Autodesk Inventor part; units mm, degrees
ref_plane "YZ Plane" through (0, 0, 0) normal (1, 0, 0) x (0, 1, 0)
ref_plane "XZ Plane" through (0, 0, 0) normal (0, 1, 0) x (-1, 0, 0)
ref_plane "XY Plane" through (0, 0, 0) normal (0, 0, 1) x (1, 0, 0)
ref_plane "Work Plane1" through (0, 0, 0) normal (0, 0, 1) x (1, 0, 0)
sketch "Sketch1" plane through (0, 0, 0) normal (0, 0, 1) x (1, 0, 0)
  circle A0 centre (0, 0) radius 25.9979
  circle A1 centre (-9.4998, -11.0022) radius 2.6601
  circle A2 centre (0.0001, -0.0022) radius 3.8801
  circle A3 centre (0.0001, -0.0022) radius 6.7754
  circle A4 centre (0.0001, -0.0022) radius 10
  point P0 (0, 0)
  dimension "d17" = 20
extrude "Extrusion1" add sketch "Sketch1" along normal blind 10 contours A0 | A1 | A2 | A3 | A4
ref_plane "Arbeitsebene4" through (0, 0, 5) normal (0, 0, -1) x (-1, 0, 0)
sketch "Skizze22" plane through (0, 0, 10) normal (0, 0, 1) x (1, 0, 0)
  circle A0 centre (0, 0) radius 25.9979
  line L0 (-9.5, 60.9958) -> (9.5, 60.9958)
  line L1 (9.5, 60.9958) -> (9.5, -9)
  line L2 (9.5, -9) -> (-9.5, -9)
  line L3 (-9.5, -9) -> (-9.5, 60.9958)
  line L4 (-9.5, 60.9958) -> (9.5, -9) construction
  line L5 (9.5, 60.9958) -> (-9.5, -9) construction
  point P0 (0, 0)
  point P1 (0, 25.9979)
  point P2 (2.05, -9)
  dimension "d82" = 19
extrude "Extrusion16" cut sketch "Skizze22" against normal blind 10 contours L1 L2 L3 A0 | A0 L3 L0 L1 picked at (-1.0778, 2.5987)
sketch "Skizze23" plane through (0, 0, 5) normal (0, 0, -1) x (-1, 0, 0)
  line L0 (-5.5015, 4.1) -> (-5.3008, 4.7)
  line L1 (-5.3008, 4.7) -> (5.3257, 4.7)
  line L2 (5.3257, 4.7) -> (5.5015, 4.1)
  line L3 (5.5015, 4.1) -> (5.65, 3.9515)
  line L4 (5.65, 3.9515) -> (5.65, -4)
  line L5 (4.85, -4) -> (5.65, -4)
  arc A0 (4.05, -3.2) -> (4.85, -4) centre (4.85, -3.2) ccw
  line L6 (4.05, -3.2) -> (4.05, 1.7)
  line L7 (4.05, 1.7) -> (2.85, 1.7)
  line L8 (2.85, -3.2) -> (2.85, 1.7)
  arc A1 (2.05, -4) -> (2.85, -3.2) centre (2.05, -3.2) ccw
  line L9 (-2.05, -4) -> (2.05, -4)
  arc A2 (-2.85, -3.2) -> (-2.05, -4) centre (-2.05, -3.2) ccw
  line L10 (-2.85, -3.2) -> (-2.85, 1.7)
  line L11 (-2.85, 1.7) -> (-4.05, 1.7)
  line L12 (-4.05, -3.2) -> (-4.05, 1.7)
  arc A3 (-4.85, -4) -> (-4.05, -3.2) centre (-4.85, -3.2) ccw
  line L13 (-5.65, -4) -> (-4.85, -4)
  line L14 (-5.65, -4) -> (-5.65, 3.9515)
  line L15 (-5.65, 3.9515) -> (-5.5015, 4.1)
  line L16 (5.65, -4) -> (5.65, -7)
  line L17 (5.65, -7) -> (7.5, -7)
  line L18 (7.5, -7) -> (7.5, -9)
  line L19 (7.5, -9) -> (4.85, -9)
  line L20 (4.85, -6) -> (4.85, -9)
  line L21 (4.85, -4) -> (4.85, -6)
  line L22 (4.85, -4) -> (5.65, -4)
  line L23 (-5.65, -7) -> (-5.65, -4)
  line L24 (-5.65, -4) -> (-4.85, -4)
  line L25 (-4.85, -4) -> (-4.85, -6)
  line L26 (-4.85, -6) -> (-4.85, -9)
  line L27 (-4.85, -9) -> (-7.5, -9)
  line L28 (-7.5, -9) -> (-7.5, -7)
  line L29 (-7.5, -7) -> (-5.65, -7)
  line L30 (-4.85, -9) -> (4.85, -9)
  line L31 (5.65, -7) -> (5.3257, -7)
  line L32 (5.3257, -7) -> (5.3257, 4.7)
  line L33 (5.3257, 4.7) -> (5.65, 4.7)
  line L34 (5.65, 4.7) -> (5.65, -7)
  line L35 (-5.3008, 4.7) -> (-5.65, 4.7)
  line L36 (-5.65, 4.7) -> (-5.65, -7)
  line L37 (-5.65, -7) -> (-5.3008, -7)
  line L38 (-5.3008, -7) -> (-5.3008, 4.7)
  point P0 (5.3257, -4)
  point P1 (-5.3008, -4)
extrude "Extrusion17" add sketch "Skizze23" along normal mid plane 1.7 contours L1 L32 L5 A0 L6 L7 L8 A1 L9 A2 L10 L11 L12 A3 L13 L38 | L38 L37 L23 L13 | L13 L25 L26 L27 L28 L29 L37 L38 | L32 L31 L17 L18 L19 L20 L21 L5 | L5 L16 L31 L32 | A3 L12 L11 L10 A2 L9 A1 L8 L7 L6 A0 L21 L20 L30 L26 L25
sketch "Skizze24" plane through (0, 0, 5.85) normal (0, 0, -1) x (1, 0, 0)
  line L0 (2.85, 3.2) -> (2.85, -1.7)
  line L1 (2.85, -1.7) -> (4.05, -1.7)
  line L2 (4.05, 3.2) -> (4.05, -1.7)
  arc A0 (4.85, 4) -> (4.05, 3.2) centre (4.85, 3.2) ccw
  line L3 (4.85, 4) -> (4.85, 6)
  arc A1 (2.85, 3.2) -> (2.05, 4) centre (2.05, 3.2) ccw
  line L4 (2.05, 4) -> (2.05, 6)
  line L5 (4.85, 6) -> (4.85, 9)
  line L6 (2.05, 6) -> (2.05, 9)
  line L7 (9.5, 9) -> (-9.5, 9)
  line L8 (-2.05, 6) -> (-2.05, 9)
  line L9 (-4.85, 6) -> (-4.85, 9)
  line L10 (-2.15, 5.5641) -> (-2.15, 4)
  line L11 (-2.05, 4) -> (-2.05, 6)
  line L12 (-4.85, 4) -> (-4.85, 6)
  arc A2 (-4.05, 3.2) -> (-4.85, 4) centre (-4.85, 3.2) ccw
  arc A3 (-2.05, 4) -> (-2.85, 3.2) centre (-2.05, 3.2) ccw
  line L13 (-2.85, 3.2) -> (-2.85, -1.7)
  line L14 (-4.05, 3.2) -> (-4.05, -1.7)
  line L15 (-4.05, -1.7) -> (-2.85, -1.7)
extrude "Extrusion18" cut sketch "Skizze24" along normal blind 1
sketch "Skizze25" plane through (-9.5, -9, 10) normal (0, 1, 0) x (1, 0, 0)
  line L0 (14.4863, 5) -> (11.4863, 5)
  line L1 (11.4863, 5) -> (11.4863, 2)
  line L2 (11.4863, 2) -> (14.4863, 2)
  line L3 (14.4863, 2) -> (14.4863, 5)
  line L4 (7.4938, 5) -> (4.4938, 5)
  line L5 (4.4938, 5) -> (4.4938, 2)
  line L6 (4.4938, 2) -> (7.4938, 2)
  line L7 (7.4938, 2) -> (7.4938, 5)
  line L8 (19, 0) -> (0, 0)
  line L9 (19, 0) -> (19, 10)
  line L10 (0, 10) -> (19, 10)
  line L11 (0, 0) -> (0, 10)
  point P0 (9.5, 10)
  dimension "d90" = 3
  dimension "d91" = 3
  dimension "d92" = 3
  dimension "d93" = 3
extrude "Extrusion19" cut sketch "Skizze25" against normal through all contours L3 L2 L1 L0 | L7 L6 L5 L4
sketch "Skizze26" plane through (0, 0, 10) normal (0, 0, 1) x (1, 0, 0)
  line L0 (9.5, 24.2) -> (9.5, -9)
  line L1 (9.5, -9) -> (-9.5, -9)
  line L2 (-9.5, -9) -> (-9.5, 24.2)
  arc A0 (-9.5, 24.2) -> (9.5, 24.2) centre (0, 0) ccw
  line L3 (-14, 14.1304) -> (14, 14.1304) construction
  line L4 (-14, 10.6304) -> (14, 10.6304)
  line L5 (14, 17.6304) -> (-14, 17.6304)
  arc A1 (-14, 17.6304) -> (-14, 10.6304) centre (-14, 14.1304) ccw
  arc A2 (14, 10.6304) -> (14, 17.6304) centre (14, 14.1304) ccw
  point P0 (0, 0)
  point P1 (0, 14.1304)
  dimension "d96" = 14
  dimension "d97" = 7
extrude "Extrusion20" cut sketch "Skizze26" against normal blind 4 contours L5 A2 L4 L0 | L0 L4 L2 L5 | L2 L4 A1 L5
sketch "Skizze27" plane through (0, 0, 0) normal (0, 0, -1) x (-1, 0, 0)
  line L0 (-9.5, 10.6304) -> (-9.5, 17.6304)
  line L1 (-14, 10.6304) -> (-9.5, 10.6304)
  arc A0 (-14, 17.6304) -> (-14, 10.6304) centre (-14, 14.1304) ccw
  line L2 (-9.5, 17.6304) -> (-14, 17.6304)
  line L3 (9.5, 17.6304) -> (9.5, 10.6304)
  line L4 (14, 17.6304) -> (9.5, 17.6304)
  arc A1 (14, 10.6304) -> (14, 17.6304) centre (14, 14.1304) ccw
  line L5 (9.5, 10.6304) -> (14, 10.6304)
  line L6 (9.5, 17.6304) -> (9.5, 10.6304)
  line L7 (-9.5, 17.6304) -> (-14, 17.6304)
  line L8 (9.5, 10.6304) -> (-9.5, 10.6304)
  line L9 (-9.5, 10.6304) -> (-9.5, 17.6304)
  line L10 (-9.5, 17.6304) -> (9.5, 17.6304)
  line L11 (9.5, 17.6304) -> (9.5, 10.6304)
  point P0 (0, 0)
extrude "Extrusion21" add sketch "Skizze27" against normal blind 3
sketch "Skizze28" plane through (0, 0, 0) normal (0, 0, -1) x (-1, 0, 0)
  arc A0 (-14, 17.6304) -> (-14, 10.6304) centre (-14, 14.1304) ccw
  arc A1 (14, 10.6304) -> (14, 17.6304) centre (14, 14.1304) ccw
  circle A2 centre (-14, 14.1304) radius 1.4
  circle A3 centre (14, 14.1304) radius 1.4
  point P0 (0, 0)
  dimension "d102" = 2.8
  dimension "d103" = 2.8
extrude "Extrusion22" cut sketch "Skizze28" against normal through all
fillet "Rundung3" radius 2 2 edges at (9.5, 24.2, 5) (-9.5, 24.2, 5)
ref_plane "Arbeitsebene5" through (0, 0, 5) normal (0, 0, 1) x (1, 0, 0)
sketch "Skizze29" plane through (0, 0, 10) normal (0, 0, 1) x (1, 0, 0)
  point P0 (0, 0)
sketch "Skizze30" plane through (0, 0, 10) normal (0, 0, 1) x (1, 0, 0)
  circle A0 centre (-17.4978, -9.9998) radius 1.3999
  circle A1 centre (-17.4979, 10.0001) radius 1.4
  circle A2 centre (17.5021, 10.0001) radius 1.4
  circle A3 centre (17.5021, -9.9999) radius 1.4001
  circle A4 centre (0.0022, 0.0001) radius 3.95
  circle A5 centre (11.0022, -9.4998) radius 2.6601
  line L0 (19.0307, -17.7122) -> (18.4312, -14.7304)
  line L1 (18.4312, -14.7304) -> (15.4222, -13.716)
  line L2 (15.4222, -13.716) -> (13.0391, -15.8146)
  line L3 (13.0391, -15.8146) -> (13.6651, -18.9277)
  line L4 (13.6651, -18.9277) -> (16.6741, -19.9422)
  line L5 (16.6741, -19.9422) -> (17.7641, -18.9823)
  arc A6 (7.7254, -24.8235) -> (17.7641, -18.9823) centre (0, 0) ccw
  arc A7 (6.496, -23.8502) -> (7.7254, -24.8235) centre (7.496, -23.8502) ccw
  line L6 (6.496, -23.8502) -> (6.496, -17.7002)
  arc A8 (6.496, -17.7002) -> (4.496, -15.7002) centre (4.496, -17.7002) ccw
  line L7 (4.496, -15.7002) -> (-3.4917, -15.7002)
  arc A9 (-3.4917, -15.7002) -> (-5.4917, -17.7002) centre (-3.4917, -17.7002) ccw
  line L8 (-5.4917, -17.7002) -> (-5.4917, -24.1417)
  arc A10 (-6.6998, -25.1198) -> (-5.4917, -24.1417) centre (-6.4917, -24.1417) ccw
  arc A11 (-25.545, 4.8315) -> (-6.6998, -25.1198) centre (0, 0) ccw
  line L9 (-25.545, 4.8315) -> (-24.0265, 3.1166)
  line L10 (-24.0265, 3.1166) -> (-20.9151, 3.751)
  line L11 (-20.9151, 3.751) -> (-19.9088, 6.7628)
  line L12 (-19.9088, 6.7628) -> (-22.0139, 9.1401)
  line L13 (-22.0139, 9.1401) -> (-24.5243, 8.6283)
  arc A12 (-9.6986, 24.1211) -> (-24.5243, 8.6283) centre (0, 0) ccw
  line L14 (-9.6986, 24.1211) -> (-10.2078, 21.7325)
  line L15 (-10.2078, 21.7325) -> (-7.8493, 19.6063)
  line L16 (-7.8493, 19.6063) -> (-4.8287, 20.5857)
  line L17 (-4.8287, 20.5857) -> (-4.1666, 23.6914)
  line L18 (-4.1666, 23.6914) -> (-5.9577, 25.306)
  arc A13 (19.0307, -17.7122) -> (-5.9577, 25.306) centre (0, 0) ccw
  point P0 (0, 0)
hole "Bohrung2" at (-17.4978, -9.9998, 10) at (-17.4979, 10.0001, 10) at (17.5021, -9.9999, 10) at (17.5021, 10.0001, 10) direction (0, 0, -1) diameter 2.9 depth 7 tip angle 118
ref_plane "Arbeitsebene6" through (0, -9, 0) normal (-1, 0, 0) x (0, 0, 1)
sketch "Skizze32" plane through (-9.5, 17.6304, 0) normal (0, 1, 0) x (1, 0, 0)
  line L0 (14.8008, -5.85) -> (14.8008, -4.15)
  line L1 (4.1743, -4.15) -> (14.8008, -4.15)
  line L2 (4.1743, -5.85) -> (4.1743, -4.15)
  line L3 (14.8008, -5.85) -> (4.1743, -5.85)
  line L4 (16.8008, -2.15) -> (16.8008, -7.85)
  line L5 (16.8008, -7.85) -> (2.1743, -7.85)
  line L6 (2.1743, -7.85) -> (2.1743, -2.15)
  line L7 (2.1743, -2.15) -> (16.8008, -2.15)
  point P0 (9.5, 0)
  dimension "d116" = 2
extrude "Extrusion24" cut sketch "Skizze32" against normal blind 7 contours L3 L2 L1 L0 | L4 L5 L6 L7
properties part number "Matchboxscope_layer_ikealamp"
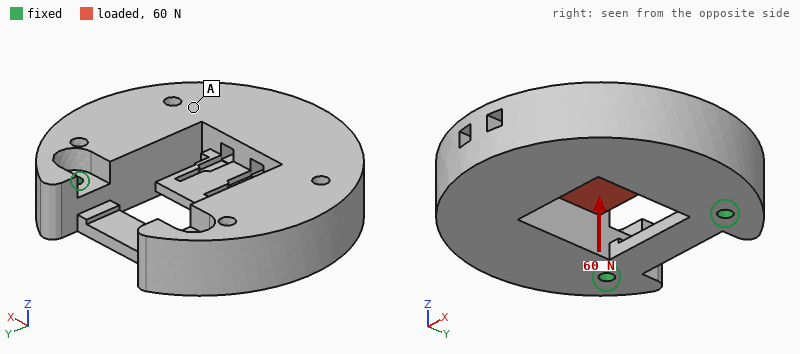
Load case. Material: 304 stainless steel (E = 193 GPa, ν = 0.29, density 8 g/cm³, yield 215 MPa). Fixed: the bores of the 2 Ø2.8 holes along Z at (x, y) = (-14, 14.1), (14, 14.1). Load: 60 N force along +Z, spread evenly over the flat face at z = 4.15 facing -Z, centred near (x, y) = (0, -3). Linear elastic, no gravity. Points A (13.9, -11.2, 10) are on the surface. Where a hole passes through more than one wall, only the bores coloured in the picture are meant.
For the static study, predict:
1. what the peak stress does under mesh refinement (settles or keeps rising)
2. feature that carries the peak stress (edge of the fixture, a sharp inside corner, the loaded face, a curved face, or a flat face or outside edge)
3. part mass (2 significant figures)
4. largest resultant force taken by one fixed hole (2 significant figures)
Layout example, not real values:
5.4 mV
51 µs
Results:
keeps rising
a sharp inside corner
110 g
30 N
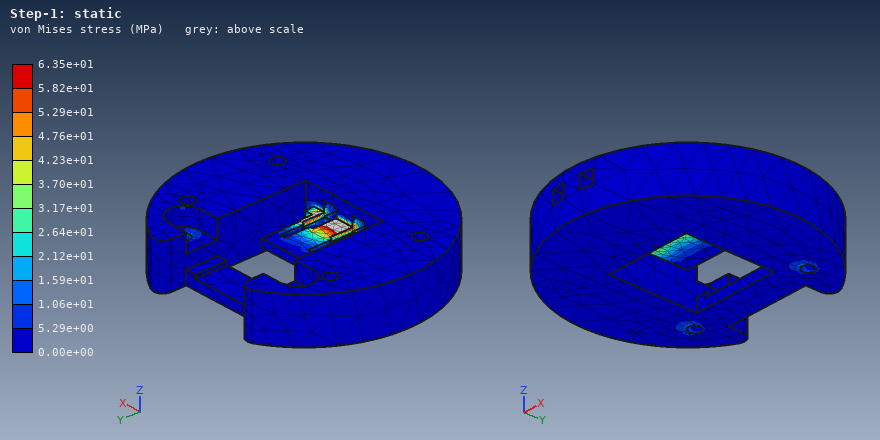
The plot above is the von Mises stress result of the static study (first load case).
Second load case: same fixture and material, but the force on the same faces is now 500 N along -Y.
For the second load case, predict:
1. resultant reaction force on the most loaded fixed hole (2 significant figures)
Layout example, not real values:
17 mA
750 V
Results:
250 N
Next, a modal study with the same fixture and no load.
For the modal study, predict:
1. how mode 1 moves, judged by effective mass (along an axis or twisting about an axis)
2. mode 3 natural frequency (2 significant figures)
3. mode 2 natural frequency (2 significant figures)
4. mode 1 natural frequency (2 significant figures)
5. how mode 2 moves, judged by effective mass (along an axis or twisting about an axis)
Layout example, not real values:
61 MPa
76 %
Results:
along Z
6000 Hz
5500 Hz
2800 Hz
along X
